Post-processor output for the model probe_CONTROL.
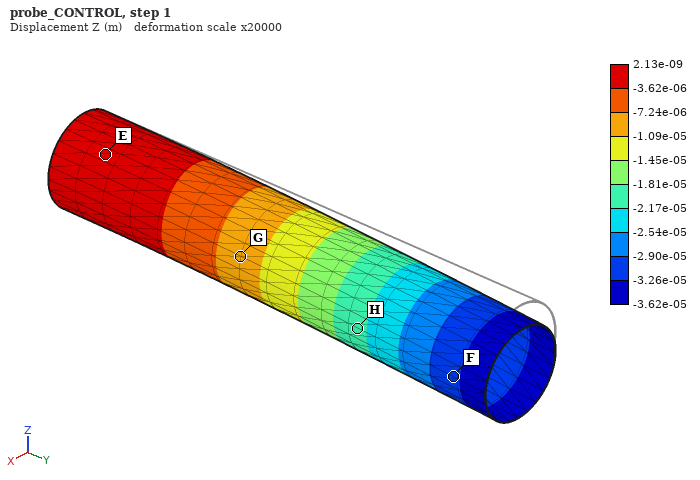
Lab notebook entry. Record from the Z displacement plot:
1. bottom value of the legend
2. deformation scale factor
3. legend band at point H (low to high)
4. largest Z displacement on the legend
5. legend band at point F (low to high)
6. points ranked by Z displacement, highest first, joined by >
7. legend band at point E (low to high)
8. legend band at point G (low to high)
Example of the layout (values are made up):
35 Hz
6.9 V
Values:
-3.62e-05 m
20000
-2.17e-05 to -1.81e-05 m
2.13e-09 m
-3.26e-05 to -2.90e-05 m
E > G > H > F
-3.62e-06 to 2.13e-09 m
-1.09e-05 to -7.24e-06 m
